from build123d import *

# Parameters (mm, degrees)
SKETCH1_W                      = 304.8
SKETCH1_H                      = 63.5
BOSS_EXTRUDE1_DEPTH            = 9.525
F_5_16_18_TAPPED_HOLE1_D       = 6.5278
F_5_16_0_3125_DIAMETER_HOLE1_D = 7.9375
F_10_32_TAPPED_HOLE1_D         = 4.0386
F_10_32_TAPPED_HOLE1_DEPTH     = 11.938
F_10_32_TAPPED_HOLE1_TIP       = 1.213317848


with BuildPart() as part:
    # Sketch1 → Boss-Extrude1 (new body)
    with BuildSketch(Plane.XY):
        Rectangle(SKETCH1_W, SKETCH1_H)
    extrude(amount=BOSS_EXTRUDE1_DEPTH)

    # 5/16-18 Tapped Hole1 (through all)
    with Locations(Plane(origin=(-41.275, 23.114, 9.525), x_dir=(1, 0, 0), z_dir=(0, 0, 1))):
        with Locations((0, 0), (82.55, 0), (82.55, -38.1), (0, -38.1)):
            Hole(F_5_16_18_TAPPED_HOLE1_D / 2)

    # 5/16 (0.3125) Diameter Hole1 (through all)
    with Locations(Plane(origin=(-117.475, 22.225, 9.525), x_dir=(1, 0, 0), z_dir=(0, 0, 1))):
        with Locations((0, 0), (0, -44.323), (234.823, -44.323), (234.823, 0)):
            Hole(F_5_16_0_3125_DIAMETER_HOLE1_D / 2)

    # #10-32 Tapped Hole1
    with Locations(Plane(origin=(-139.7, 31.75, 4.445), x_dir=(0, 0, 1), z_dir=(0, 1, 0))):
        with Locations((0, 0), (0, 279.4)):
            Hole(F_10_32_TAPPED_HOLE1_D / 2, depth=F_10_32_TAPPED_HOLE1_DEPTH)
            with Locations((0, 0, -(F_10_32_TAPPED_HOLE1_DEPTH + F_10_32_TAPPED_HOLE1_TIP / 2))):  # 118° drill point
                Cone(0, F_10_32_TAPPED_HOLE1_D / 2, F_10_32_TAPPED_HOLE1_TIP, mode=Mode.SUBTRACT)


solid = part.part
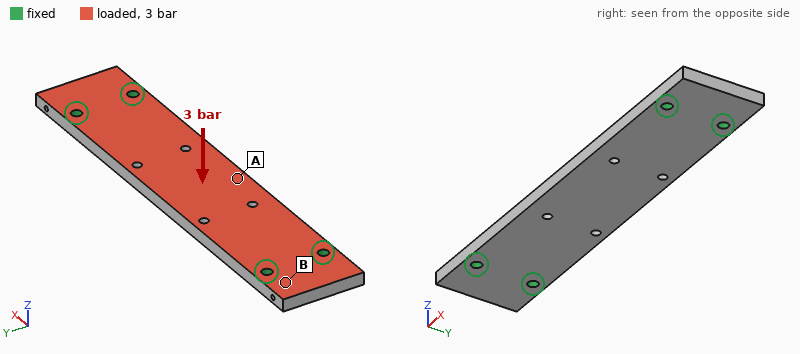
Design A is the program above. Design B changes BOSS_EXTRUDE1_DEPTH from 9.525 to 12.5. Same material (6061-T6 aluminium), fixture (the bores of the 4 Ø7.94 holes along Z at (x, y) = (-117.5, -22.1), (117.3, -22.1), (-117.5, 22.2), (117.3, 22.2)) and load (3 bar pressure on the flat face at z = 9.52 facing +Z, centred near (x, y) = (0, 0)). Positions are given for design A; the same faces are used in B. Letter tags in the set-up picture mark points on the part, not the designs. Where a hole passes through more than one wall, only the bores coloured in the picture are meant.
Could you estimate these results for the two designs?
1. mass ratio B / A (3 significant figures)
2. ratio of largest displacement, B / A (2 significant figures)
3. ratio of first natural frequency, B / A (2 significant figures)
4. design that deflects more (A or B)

1.31
0.46
1.3
A
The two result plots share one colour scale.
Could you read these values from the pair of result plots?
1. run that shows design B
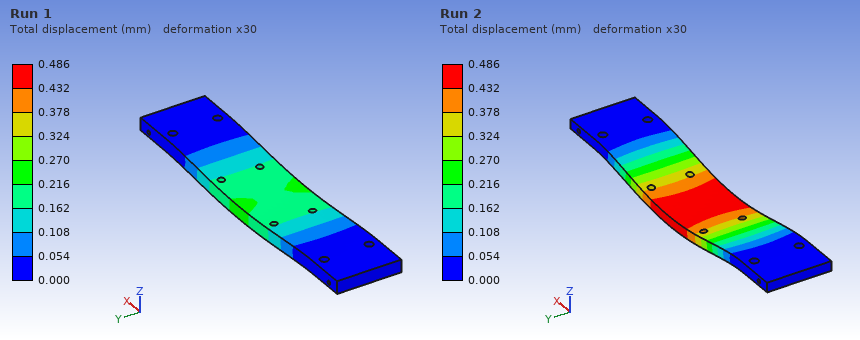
Run 1
